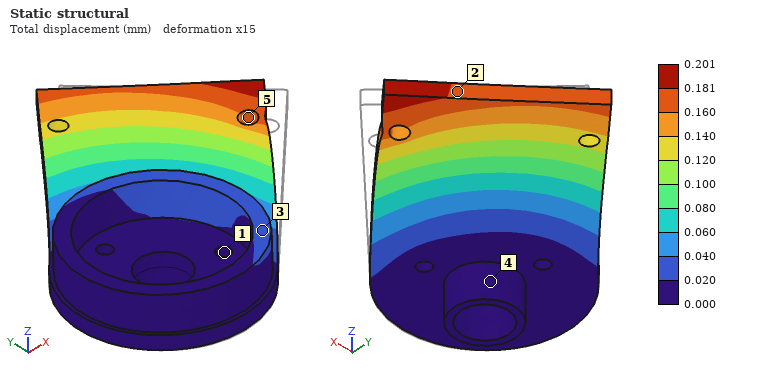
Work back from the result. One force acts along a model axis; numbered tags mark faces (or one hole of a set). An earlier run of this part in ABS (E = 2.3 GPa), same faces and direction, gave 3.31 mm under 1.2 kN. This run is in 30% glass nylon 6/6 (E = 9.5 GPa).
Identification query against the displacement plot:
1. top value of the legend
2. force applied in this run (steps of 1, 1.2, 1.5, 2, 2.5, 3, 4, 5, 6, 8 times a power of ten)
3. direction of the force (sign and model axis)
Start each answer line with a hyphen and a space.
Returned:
- 0.201 mm
- 300 N
- +Y
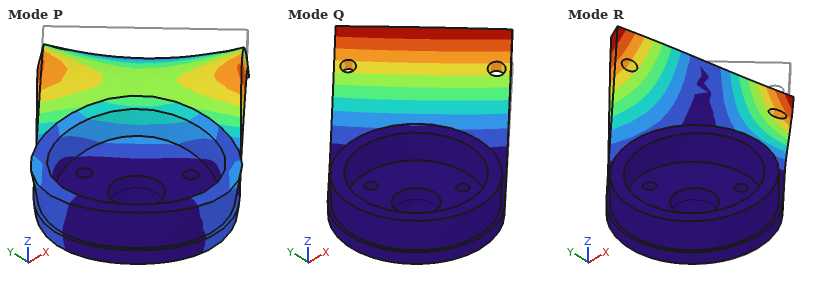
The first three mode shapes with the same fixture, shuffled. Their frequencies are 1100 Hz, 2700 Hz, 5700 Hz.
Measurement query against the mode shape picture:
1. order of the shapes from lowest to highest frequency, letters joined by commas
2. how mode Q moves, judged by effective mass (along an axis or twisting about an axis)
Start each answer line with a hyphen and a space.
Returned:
- Q, R, P
- along Z
